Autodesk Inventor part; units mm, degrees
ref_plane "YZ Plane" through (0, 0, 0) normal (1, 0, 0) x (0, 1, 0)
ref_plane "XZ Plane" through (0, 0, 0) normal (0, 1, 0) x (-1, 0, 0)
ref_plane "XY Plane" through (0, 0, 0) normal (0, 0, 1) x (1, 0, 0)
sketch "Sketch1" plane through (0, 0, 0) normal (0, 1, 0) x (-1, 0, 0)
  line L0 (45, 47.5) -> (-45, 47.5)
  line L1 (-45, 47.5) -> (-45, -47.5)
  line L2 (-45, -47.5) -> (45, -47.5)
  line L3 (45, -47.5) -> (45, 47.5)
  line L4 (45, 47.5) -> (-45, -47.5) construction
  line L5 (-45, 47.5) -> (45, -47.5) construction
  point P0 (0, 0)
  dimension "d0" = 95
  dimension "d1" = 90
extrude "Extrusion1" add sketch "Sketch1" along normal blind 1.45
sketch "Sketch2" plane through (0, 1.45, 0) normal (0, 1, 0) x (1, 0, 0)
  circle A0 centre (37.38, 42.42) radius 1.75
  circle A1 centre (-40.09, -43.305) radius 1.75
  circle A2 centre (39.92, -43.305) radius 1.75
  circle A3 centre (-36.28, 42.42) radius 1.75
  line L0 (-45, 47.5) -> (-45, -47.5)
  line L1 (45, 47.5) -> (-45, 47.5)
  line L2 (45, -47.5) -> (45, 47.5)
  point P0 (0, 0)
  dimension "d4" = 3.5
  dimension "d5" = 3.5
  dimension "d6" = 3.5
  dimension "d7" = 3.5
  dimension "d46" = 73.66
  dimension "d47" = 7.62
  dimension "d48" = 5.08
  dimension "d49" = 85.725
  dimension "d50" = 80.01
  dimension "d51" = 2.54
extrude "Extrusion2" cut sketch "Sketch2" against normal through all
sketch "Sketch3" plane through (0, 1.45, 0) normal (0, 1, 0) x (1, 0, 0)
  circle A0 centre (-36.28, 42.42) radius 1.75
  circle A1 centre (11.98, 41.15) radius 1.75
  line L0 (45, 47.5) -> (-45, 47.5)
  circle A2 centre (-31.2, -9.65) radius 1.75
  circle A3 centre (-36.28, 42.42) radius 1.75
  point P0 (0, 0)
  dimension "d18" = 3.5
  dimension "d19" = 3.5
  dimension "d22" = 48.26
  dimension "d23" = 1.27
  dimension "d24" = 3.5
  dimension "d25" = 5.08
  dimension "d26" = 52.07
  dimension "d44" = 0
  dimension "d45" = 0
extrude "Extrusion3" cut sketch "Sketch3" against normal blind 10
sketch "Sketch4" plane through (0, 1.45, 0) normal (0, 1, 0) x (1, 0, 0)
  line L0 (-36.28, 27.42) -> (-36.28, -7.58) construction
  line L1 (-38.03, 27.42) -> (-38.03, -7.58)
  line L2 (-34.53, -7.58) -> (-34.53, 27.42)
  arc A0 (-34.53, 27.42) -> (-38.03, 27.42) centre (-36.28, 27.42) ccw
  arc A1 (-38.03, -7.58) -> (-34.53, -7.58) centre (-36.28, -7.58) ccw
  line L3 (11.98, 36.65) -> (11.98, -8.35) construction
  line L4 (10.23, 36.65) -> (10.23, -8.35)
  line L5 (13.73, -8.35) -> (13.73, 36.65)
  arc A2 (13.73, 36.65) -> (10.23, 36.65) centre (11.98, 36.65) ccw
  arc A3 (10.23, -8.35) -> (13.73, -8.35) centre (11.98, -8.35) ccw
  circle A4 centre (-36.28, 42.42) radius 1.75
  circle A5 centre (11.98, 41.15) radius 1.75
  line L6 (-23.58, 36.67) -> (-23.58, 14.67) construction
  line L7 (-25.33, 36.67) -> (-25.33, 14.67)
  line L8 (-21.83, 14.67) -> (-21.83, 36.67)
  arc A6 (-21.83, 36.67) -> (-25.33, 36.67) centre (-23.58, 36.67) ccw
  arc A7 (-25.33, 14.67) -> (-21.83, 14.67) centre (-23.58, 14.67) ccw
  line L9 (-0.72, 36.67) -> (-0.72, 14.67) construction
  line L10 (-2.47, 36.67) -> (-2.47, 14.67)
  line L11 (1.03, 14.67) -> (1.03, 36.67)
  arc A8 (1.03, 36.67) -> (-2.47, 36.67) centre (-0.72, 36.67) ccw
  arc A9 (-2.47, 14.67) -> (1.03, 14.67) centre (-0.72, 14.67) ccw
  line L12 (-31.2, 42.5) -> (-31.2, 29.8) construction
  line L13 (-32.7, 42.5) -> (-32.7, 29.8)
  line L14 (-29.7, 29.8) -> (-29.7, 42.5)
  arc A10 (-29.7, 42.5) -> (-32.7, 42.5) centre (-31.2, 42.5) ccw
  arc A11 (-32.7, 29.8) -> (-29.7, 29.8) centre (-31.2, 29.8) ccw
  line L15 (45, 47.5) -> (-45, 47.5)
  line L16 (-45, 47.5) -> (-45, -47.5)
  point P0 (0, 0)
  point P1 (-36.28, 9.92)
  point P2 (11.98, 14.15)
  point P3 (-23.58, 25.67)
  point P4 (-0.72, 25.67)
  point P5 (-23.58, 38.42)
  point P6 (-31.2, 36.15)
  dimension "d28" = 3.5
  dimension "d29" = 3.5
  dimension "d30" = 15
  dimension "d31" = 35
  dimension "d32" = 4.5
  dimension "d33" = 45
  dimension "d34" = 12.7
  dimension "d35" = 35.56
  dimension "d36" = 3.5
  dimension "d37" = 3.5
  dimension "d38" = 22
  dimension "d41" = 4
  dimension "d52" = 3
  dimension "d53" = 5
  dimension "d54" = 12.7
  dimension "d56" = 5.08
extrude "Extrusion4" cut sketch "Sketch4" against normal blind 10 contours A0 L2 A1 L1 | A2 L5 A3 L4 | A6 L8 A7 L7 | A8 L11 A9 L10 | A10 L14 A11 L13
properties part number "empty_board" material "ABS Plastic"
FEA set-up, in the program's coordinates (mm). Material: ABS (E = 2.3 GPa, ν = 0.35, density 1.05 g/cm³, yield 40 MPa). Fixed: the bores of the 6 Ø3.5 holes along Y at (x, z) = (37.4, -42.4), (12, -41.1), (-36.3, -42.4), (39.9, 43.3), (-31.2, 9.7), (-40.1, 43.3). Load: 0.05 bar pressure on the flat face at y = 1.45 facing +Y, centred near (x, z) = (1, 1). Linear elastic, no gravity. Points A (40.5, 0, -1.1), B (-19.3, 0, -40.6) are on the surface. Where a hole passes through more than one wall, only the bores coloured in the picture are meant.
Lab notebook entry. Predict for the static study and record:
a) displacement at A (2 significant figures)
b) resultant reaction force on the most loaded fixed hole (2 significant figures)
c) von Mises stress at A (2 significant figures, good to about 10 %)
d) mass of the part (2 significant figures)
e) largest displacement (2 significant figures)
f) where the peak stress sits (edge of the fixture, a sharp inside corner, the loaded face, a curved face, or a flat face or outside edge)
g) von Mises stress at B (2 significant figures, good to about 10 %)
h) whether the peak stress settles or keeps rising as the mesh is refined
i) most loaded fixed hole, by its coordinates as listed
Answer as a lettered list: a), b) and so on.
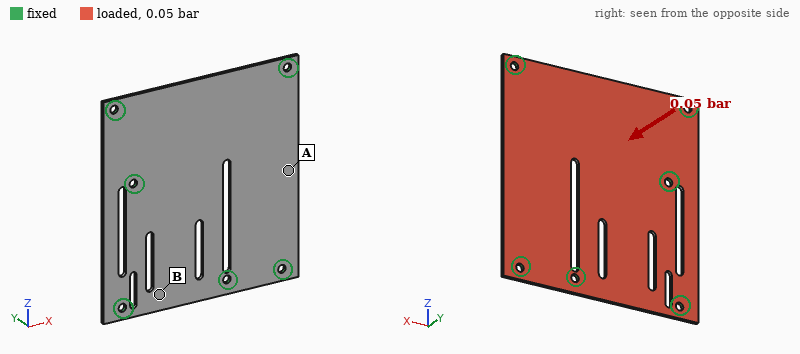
a) 1.2 mm
b) 12 N
c) 4.4 MPa
d) 12 g
e) 1.4 mm
f) edge of the fixture
g) 1.7 MPa
h) keeps rising
i) (-31.2, 9.7)
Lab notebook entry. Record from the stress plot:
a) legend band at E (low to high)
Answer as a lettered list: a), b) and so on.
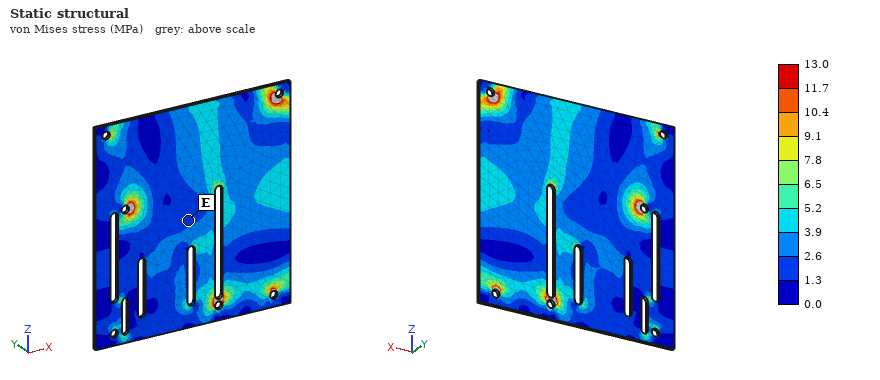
a) 1.3 to 2.6 MPa
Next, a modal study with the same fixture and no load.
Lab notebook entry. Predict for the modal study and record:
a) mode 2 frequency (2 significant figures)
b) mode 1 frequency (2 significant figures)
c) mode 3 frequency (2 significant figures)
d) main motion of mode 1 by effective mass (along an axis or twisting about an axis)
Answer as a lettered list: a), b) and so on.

a) 400 Hz
b) 290 Hz
c) 500 Hz
d) along Y
